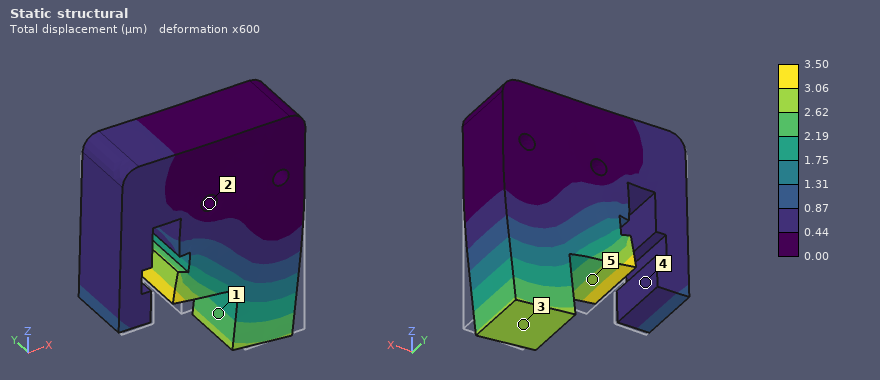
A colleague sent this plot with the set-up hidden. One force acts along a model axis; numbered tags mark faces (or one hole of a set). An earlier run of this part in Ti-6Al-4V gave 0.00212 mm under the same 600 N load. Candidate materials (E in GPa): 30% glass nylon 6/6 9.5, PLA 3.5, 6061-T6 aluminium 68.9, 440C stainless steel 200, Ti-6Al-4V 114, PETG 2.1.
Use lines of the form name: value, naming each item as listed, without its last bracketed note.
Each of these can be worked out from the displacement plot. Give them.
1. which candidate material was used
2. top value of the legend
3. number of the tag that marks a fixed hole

which candidate material was used: 6061-T6 aluminium
top value of the legend: 3.50 µm
number of the tag that marks a fixed hole: 2
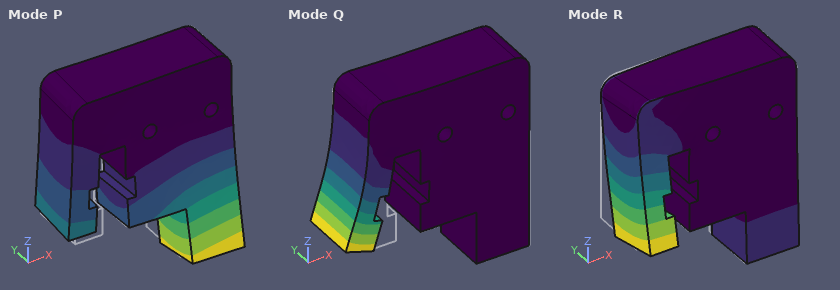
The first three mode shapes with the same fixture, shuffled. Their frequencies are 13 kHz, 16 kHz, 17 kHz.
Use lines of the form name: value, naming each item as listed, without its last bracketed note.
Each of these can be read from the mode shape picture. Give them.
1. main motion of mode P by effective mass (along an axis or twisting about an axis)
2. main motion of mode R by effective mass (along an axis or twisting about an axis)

main motion of mode P by effective mass: along Y
main motion of mode R by effective mass: along Y
